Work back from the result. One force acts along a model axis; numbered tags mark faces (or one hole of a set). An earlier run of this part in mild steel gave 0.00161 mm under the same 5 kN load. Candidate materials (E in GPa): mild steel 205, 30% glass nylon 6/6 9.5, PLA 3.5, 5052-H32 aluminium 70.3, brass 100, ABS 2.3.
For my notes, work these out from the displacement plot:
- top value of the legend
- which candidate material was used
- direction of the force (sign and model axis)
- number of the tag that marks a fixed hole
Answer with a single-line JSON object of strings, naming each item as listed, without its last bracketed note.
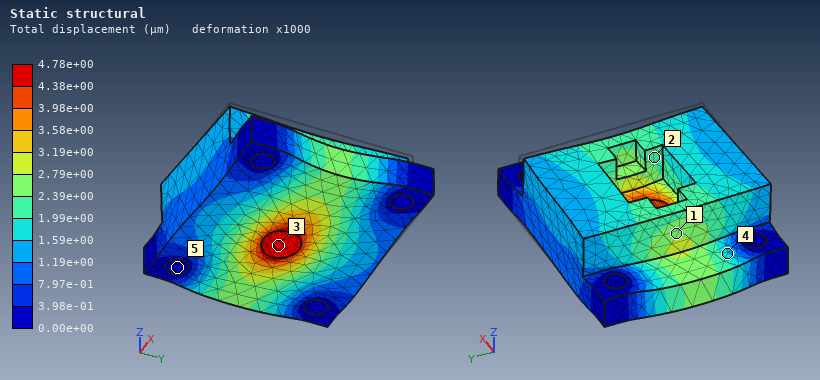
{"top value of the legend": "4.78e+00 µm", "which candidate material was used": "5052-H32 aluminium", "direction of the force": "-X", "number of the tag that marks a fixed hole": "5"}
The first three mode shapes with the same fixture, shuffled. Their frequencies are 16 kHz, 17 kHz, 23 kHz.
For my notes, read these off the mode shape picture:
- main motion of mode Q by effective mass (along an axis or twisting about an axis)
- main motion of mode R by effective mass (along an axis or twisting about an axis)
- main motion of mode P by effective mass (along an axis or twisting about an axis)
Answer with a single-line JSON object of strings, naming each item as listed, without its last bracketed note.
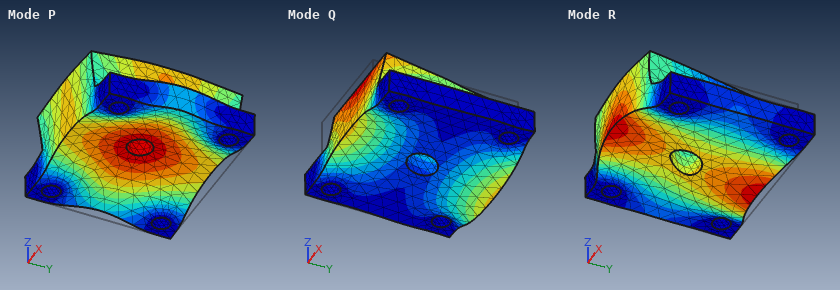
{"main motion of mode Q by effective mass": "along Y", "main motion of mode R by effective mass": "along Y", "main motion of mode P by effective mass": "along Z"}
